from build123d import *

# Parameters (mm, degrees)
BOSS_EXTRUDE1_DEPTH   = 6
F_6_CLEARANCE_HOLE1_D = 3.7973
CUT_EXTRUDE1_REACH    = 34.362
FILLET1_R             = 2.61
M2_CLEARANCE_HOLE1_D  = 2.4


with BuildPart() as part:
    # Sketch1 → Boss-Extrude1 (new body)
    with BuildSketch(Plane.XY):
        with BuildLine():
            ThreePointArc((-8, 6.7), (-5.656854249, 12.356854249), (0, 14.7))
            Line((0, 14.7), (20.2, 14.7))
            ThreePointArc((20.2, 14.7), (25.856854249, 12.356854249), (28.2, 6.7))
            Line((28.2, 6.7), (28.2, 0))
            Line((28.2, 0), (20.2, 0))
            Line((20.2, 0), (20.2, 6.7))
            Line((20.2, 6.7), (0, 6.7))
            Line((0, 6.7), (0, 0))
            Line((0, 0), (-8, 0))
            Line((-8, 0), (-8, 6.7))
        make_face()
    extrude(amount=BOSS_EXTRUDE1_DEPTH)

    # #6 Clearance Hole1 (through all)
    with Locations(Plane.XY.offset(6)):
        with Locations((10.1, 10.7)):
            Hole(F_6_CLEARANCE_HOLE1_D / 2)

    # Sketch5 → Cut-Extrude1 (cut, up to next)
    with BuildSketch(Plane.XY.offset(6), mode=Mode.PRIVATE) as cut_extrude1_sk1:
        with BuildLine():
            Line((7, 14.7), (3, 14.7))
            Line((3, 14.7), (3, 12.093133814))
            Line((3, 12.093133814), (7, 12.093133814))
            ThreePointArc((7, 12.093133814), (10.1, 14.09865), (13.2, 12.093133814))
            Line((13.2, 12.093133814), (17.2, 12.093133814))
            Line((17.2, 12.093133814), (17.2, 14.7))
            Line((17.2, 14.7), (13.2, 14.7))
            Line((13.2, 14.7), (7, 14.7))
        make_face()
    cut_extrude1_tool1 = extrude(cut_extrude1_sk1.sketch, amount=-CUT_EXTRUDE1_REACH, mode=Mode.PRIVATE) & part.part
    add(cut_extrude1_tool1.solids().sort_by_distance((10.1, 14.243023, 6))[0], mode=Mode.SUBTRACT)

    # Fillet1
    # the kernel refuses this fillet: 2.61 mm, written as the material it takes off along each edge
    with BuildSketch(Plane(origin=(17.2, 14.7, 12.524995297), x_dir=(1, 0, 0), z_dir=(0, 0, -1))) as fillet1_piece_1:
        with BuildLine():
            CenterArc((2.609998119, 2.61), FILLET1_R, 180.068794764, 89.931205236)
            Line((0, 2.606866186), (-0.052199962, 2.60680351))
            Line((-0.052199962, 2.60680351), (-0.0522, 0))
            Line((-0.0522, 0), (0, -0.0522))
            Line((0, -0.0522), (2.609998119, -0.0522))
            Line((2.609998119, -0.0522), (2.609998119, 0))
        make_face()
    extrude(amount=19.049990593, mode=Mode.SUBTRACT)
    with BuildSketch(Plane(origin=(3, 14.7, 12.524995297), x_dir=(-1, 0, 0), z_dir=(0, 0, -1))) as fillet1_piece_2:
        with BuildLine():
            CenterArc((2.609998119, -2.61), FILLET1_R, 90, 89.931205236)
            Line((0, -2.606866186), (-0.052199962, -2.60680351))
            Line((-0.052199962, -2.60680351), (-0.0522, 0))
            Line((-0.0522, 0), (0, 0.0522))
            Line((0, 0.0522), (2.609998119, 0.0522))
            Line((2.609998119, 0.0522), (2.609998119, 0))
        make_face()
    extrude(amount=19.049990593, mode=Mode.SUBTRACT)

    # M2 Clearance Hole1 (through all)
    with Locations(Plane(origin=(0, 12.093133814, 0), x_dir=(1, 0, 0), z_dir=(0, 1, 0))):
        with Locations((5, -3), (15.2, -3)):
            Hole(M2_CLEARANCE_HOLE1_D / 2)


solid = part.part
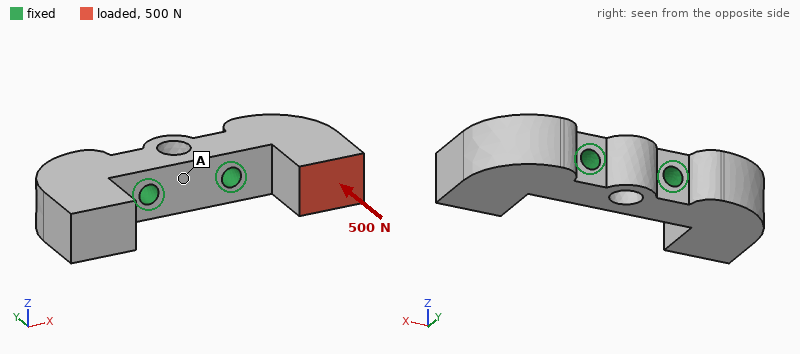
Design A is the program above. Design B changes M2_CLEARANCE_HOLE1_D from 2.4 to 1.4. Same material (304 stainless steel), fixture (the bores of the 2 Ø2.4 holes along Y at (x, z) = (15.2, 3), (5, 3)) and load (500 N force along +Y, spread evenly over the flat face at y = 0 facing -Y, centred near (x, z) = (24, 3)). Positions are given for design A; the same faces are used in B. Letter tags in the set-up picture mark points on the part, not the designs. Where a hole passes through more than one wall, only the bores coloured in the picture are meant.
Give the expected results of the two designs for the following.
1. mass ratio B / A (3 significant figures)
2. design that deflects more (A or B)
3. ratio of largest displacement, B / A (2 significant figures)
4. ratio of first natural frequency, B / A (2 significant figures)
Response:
1.02
B
1.3
0.84
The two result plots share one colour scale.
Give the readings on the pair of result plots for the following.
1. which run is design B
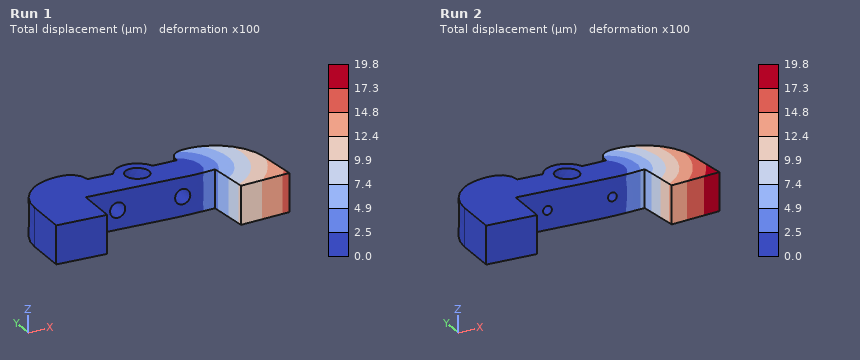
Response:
Run 2
